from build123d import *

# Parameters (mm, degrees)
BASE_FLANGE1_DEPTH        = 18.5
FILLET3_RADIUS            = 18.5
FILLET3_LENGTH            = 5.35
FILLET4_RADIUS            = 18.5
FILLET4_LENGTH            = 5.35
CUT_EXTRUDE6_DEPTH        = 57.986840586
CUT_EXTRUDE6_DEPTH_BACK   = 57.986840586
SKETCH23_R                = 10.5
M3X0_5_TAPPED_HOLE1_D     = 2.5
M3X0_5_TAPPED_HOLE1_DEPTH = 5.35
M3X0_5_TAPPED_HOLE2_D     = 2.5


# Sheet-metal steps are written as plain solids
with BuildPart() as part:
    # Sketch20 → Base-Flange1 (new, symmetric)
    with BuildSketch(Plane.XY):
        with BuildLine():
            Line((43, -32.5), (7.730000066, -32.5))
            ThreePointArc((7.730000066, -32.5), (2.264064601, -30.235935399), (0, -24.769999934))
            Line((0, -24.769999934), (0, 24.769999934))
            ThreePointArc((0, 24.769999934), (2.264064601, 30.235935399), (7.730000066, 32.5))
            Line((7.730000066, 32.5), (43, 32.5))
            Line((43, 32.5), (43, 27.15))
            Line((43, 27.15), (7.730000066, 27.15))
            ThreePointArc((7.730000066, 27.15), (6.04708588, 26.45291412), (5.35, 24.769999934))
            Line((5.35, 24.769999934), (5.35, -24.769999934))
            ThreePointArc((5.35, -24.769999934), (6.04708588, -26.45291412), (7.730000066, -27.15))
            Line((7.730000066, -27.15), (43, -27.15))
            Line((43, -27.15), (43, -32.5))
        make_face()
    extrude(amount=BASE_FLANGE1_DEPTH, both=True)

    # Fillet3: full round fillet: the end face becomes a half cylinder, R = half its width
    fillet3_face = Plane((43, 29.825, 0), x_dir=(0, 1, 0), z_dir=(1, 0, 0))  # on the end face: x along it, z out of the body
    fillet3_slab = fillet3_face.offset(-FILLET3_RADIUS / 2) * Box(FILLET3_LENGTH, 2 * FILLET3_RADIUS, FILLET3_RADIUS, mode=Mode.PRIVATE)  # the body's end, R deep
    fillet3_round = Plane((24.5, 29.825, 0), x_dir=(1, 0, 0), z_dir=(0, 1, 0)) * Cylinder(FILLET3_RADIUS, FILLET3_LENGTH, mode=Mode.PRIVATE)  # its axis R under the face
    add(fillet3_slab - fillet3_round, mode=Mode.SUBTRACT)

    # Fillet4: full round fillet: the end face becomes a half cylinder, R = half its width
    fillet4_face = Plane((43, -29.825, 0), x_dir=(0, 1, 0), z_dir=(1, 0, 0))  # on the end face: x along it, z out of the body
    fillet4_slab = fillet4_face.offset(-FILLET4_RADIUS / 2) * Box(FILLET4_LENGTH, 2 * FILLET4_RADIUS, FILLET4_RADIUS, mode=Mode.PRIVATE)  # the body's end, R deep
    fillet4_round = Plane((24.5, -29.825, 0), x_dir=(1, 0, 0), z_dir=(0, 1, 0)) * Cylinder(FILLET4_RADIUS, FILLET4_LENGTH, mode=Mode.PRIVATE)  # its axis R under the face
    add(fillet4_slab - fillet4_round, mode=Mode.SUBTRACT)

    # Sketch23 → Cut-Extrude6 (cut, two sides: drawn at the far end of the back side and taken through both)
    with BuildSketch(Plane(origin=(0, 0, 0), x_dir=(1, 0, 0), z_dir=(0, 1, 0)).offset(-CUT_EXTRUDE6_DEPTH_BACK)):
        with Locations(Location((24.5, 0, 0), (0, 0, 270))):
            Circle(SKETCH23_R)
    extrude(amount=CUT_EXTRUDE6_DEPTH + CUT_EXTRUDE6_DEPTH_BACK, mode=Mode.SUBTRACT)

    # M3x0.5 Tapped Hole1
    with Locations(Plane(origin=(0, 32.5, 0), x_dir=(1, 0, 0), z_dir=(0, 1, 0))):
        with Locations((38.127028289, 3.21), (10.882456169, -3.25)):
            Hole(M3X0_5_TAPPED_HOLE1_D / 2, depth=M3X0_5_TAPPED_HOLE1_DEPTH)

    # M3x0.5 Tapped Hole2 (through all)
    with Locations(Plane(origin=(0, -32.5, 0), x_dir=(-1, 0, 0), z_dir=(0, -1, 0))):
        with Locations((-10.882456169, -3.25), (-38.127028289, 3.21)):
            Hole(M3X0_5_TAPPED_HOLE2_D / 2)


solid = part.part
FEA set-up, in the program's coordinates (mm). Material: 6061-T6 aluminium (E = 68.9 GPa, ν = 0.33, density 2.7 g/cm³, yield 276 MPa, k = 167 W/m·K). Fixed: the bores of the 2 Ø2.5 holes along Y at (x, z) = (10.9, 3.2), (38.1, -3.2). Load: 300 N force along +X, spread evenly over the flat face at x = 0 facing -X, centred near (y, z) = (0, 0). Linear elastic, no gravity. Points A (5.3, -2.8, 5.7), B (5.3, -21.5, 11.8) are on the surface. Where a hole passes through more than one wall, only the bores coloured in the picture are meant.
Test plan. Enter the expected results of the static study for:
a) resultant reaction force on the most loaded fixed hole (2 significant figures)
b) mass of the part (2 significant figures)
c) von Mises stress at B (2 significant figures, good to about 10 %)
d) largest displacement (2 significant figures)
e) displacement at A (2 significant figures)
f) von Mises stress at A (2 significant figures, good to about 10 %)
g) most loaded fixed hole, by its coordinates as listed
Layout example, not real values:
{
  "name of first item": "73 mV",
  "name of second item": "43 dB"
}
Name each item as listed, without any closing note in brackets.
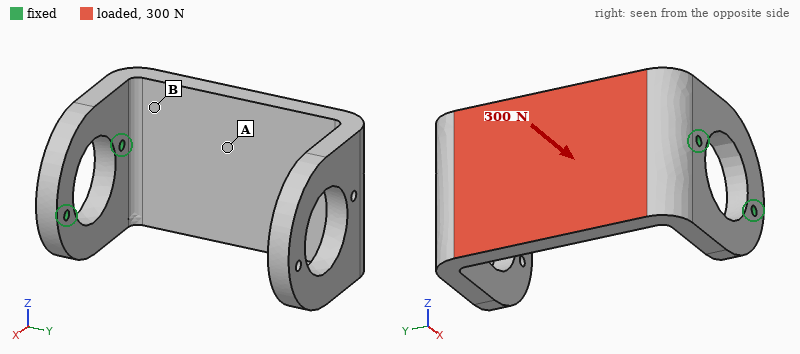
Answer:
{
  "resultant reaction force on the most loaded fixed hole": "310 N",
  "mass of the part": "58 g",
  "von Mises stress at B": "37 MPa",
  "largest displacement": "0.51 mm",
  "displacement at A": "0.15 mm",
  "von Mises stress at A": "12 MPa",
  "most loaded fixed hole, by its coordinates as listed": "(10.9, 3.2)"
}
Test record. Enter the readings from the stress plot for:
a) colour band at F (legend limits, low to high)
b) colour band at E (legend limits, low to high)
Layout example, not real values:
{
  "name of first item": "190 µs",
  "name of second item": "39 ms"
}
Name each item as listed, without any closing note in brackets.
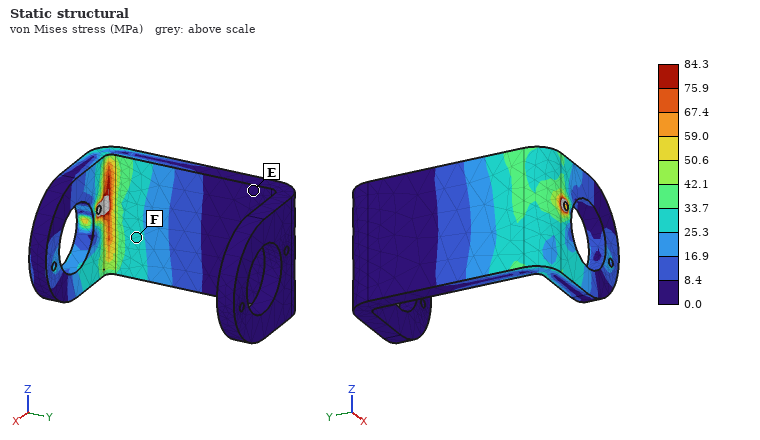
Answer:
{
  "colour band at F": "25.3 to 33.7 MPa",
  "colour band at E": "0.0 to 8.4 MPa"
}
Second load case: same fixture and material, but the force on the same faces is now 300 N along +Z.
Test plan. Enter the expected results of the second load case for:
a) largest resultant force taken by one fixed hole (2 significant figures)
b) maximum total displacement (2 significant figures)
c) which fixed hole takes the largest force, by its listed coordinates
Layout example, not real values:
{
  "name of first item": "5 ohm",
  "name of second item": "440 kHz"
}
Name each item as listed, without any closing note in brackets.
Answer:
{
  "largest resultant force taken by one fixed hole": "380 N",
  "maximum total displacement": "0.20 mm",
  "which fixed hole takes the largest force, by its listed coordinates": "(10.9, 3.2)"
}
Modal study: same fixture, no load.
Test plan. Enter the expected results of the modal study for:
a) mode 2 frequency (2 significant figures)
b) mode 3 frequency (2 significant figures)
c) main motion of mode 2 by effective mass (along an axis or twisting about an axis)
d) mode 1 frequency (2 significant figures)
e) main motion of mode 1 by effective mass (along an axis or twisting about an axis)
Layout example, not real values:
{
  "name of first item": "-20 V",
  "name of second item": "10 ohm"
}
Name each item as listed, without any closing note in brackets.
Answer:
{
  "mode 2 frequency": "820 Hz",
  "mode 3 frequency": "1900 Hz",
  "main motion of mode 2 by effective mass": "along Z",
  "mode 1 frequency": "560 Hz",
  "main motion of mode 1 by effective mass": "along X"
}
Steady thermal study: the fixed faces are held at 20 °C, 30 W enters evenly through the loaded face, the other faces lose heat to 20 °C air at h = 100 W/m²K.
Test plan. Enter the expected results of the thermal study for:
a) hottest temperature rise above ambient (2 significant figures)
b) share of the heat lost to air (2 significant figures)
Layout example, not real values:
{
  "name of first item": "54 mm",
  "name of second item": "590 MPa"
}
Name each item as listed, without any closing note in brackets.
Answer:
{
  "hottest temperature rise above ambient": "22 K",
  "share of the heat lost to air": "39 %"
}
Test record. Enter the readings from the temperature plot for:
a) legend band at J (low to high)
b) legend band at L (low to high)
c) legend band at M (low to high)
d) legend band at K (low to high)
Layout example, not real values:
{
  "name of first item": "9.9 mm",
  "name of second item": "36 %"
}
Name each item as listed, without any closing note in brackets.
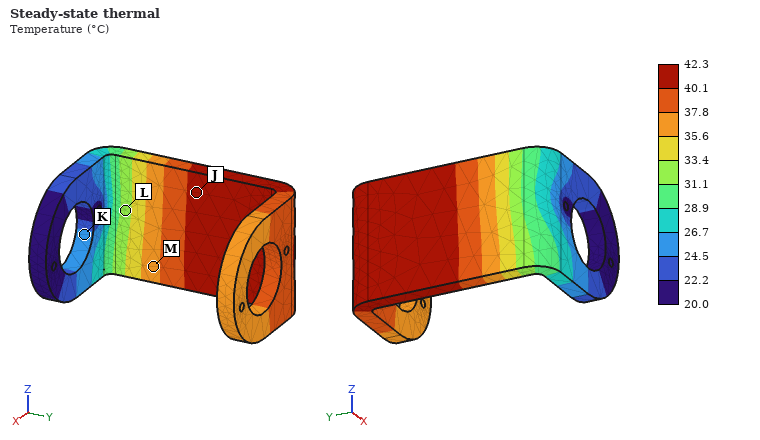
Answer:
{
  "legend band at J": "40.1 to 42.3 °C",
  "legend band at L": "31.1 to 33.4 °C",
  "legend band at M": "35.6 to 37.8 °C",
  "legend band at K": "24.5 to 26.7 °C"
}
